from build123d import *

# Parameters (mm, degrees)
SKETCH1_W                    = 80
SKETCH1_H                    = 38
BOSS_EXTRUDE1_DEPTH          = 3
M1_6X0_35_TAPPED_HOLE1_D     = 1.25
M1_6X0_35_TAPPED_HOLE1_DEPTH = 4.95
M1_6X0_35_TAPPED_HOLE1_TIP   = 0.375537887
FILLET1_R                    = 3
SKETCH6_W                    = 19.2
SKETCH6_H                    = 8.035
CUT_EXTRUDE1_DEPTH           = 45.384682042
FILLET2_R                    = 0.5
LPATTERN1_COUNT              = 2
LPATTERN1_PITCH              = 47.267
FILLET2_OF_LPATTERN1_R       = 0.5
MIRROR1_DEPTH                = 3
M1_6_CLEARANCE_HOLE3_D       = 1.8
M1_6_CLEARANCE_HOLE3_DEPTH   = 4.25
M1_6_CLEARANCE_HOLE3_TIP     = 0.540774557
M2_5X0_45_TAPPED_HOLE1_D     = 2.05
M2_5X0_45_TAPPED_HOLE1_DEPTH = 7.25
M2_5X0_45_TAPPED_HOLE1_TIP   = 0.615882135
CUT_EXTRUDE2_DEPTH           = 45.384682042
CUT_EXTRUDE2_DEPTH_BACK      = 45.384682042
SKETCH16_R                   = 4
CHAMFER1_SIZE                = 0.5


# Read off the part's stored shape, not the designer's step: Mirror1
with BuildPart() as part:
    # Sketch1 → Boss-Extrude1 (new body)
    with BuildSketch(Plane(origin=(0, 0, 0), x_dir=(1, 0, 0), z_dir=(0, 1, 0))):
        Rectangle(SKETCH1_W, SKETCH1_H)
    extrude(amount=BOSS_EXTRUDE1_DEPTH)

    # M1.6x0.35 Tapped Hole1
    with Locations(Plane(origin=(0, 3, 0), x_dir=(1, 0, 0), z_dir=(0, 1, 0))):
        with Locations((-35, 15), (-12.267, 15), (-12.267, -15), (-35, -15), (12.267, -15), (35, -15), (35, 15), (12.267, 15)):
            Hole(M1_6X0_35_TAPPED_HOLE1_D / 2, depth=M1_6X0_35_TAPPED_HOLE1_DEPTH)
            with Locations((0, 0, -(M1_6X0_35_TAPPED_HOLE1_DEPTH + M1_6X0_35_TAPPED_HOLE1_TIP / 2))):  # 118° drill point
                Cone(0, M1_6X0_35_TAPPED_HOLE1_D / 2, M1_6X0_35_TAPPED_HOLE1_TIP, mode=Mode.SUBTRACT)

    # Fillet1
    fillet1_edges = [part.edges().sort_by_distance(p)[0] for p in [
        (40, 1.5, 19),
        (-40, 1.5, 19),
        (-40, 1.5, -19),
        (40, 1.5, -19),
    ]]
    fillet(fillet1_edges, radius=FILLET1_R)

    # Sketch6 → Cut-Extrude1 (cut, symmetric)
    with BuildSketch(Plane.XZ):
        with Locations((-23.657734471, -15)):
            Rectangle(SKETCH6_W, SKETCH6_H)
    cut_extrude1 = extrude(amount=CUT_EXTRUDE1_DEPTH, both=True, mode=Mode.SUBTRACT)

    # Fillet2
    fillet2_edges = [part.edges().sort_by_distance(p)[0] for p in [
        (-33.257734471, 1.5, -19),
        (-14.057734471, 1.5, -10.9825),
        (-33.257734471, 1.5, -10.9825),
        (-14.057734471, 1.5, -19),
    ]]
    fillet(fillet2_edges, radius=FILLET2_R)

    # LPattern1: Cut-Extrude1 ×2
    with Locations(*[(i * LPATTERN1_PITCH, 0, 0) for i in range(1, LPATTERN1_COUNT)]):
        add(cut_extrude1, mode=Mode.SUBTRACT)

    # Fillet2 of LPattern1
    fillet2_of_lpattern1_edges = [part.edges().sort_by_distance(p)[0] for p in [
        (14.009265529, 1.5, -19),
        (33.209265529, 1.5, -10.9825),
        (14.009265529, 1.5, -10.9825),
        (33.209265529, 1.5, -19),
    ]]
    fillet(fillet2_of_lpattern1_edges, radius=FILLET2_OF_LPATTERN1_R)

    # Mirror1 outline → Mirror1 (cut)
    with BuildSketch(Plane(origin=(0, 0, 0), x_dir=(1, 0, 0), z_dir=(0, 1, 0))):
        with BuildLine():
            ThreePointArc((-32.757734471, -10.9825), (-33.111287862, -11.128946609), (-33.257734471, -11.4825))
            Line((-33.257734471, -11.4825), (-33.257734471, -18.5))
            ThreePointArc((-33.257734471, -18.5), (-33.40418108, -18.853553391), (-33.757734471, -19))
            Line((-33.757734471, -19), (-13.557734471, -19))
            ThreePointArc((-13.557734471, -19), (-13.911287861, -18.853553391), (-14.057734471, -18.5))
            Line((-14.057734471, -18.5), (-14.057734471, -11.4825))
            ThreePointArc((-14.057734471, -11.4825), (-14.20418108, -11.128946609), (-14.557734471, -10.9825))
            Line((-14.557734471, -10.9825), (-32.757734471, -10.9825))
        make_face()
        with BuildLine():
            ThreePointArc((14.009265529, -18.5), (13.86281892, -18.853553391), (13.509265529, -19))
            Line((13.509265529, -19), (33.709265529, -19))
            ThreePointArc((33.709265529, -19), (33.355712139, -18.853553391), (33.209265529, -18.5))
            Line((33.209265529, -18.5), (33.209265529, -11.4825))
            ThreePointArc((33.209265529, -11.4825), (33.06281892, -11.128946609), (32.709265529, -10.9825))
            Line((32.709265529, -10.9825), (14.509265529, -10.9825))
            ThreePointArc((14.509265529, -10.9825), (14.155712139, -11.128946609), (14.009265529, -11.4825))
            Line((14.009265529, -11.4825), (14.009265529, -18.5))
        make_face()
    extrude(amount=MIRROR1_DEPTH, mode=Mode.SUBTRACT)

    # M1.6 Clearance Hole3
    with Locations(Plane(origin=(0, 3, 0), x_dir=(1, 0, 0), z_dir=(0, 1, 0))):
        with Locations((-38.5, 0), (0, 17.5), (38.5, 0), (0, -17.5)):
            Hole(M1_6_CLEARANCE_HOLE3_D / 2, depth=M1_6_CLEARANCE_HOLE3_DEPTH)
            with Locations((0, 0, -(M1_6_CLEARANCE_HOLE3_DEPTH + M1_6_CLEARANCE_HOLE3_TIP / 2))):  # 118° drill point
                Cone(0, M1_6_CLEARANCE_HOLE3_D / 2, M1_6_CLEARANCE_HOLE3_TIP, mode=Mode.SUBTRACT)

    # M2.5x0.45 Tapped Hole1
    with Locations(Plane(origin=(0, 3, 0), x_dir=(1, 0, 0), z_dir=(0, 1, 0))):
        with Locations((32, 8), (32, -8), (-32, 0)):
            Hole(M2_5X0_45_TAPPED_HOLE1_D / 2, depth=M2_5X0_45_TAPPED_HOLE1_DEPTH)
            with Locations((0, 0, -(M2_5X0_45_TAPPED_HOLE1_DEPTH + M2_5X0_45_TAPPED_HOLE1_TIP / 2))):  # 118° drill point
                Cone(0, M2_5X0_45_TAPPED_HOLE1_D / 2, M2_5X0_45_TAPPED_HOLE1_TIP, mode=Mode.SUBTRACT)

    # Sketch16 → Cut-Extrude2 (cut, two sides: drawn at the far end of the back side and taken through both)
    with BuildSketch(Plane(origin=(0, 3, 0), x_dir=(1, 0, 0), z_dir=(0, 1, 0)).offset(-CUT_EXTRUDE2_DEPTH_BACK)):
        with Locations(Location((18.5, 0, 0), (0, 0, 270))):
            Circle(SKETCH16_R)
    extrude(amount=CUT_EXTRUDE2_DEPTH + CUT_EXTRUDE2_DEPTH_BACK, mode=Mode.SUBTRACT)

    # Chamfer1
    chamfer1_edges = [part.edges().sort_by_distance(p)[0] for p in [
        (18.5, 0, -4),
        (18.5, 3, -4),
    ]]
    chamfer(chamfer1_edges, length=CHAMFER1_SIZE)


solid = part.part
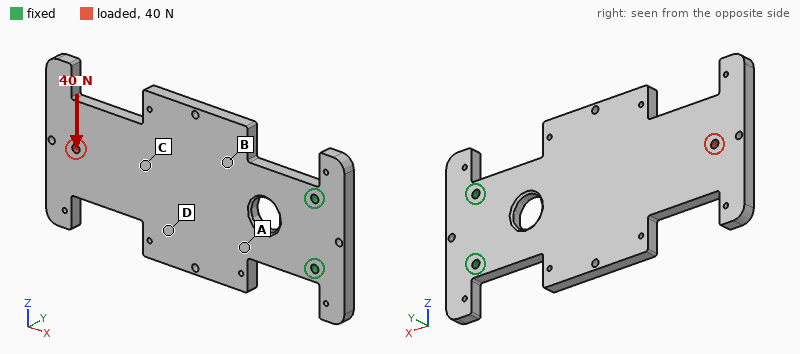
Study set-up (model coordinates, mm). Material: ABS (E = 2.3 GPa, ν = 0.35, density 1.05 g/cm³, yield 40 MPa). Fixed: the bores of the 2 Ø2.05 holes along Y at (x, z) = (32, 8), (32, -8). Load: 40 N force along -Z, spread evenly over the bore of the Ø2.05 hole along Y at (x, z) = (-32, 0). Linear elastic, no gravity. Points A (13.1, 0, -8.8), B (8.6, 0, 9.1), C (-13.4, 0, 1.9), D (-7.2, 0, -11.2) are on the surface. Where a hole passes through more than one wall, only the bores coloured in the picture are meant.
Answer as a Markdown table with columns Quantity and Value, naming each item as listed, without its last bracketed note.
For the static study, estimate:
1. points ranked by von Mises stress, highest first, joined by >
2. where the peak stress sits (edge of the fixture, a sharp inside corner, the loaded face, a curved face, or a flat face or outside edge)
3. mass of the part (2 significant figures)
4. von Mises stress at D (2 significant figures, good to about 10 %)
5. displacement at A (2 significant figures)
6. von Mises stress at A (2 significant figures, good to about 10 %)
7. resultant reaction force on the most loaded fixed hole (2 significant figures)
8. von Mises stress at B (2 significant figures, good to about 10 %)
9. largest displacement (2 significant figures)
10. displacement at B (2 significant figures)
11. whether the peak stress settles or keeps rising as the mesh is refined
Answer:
| Quantity | Value |
|---|---|
| points ranked by von Mises stress, highest first, joined by > | A > B > D > C |
| where the peak stress sits | edge of the fixture |
| mass of the part | 7.4 g |
| von Mises stress at D | 1.8 MPa |
| displacement at A | 0.12 mm |
| von Mises stress at A | 4.4 MPa |
| resultant reaction force on the most loaded fixed hole | 160 N |
| von Mises stress at B | 3.3 MPa |
| largest displacement | 0.69 mm |
| displacement at B | 0.17 mm |
| whether the peak stress settles or keeps rising as the mesh is refined | keeps rising |
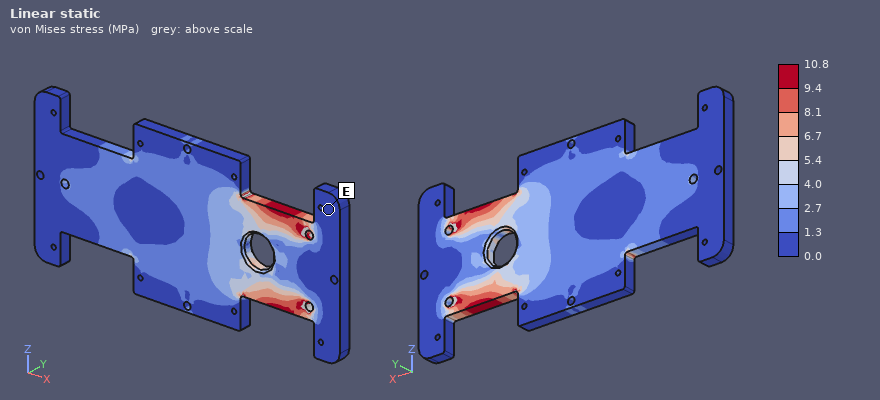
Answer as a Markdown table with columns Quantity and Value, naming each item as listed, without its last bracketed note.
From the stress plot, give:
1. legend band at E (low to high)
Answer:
| Quantity | Value |
|---|---|
| legend band at E | 0.0 to 1.3 MPa |
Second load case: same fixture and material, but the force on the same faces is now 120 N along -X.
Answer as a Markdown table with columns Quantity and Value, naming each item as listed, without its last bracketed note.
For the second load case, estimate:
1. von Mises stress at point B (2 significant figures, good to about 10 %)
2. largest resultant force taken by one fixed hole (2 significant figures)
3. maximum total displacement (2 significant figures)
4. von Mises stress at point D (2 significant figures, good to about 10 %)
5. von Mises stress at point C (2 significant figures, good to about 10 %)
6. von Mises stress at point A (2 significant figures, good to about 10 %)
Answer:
| Quantity | Value |
|---|---|
| von Mises stress at point B | 1.8 MPa |
| largest resultant force taken by one fixed hole | 60 N |
| maximum total displacement | 65 µm |
| von Mises stress at point D | 1.2 MPa |
| von Mises stress at point C | 1.6 MPa |
| von Mises stress at point A | 2.1 MPa |
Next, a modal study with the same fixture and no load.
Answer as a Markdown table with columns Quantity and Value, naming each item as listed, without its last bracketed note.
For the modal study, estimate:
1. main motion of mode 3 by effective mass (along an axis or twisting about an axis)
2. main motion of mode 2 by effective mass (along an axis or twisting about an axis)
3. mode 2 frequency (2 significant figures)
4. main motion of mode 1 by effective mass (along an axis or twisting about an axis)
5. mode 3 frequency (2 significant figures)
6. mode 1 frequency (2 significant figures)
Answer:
| Quantity | Value |
|---|---|
| main motion of mode 3 by effective mass | along Y |
| main motion of mode 2 by effective mass | twisting about X |
| mode 2 frequency | 520 Hz |
| main motion of mode 1 by effective mass | along Y |
| mode 3 frequency | 730 Hz |
| mode 1 frequency | 110 Hz |
